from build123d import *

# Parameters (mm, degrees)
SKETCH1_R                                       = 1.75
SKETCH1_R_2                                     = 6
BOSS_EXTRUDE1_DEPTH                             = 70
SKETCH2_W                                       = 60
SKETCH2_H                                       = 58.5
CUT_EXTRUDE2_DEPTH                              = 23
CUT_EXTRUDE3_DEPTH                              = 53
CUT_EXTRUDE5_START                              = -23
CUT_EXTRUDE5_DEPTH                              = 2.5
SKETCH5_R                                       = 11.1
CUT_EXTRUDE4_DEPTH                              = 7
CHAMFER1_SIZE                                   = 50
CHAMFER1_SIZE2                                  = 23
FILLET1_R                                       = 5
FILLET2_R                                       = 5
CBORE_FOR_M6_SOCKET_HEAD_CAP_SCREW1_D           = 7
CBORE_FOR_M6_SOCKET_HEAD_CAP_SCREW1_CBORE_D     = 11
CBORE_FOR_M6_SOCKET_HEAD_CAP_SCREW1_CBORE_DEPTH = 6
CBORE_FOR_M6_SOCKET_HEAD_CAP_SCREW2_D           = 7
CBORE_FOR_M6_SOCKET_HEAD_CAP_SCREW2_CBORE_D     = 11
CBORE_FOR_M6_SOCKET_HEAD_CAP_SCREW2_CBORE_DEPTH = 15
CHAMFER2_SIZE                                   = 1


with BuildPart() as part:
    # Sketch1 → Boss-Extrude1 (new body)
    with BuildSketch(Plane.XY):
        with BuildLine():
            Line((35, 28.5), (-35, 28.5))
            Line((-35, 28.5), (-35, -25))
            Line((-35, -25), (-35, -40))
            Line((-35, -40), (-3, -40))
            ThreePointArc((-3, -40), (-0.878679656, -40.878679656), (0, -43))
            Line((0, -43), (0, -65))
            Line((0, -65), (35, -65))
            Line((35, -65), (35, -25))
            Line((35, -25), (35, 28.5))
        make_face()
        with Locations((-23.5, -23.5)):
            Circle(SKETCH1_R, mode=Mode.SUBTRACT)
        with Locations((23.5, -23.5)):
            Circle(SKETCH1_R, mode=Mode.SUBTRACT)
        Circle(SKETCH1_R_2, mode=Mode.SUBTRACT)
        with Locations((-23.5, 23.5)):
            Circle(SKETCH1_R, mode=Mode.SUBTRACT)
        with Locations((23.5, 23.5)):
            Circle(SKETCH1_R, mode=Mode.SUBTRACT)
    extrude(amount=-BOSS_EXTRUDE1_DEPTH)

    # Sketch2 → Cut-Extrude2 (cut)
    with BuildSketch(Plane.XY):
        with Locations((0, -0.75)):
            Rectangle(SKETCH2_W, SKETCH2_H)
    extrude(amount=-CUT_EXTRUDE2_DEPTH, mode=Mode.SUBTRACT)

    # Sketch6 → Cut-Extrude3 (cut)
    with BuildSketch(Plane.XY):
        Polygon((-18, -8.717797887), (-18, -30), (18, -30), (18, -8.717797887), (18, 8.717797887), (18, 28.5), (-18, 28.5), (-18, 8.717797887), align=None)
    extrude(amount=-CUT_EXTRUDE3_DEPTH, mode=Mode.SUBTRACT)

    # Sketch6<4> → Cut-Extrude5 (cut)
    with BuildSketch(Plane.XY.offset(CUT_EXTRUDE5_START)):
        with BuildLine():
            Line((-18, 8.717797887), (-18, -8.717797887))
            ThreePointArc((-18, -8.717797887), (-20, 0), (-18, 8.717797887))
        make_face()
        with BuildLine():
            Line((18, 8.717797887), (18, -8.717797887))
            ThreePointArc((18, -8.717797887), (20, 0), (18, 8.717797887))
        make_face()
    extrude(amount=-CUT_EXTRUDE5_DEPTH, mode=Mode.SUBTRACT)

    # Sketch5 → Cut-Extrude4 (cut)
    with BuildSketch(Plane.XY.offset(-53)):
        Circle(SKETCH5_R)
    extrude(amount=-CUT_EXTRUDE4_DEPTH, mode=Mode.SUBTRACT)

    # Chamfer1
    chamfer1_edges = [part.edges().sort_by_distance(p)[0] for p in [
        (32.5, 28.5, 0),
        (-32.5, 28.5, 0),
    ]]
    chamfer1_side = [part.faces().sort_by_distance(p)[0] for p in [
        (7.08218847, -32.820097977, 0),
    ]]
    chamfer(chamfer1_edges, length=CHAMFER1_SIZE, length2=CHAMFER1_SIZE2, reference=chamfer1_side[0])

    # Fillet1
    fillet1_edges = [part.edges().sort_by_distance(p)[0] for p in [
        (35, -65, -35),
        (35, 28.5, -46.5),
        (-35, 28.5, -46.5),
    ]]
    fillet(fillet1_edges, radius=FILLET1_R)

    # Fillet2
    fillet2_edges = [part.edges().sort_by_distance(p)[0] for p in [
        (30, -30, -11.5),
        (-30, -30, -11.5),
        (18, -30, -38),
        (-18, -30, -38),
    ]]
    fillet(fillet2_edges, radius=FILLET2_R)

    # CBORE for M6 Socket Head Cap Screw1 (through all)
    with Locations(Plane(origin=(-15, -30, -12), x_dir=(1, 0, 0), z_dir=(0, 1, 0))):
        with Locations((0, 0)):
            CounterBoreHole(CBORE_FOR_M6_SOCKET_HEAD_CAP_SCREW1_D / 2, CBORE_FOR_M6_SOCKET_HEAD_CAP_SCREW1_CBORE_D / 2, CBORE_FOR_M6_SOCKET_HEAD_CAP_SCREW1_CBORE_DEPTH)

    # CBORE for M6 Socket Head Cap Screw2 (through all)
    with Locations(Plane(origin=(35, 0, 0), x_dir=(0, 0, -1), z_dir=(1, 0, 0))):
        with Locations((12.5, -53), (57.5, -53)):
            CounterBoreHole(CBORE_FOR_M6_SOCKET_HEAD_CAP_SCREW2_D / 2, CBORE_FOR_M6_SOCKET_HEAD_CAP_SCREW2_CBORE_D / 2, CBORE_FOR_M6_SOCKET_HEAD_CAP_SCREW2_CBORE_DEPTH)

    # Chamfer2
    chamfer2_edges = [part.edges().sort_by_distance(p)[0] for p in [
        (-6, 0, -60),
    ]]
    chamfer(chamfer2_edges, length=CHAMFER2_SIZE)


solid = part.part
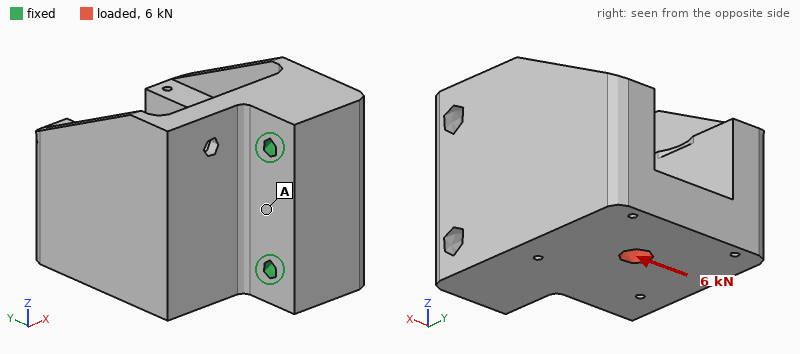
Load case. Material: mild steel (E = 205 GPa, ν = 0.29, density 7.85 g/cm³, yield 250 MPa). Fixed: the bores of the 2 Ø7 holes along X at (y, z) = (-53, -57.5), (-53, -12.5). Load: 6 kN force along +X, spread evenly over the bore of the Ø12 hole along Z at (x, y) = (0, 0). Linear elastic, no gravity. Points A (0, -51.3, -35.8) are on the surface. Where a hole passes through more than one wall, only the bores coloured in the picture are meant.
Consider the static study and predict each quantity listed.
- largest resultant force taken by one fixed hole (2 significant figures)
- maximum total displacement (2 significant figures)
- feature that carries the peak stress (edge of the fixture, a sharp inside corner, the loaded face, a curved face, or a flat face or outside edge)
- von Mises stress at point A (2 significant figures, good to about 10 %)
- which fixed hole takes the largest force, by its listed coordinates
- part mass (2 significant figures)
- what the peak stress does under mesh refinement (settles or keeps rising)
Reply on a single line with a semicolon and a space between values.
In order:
6.3 kN; 54 µm; edge of the fixture; 13 MPa; (-53, -57.5); 1.9 kg; keeps rising
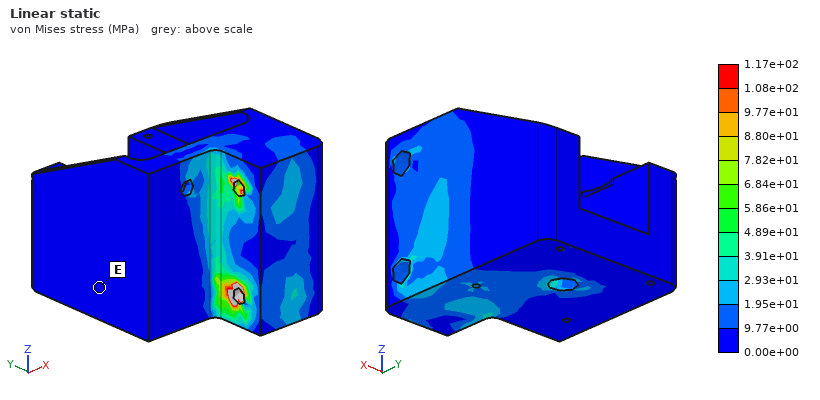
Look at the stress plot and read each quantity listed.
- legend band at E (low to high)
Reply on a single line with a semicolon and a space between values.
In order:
0.00e+00 to 9.77e+00 MPa
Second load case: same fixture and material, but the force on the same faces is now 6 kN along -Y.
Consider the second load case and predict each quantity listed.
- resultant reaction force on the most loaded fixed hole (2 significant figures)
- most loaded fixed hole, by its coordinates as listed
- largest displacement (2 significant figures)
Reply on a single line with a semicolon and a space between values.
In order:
6.9 kN; (-53, -57.5); 16 µm
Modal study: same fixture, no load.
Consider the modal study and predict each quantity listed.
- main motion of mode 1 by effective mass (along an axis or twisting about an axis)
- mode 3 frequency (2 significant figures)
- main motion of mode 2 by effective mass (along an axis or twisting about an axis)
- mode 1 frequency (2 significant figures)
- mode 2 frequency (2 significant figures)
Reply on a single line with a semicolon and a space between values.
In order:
along X; 5900 Hz; along Z; 1800 Hz; 3300 Hz
